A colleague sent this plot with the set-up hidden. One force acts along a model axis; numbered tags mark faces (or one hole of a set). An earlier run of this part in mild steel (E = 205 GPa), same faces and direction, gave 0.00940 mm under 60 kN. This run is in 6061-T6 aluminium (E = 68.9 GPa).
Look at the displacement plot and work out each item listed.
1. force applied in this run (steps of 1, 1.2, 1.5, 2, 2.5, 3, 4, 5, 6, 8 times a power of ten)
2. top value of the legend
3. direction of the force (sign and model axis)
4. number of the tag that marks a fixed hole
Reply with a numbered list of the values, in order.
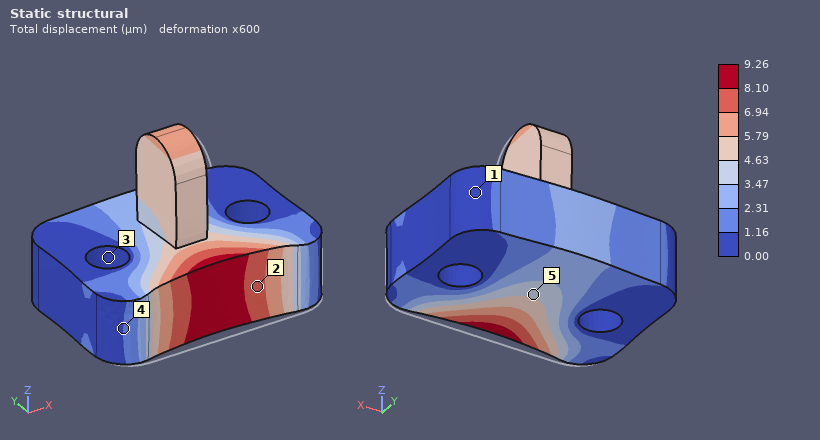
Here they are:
1. 20 kN
2. 9.26 µm
3. +Y
4. 3
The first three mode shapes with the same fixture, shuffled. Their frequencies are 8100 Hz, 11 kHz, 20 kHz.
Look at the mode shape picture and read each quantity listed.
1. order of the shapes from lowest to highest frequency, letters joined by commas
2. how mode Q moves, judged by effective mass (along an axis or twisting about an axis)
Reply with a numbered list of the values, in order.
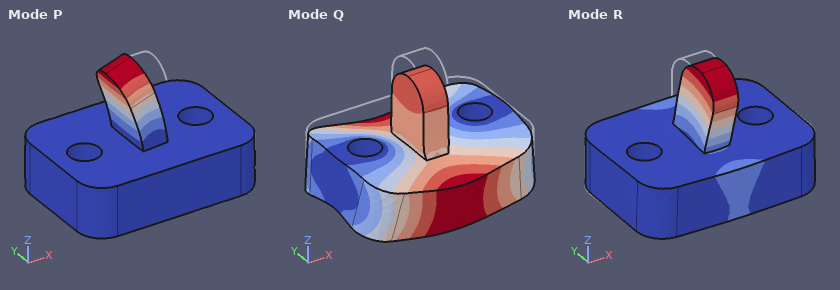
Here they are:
1. P, R, Q
2. along Z
